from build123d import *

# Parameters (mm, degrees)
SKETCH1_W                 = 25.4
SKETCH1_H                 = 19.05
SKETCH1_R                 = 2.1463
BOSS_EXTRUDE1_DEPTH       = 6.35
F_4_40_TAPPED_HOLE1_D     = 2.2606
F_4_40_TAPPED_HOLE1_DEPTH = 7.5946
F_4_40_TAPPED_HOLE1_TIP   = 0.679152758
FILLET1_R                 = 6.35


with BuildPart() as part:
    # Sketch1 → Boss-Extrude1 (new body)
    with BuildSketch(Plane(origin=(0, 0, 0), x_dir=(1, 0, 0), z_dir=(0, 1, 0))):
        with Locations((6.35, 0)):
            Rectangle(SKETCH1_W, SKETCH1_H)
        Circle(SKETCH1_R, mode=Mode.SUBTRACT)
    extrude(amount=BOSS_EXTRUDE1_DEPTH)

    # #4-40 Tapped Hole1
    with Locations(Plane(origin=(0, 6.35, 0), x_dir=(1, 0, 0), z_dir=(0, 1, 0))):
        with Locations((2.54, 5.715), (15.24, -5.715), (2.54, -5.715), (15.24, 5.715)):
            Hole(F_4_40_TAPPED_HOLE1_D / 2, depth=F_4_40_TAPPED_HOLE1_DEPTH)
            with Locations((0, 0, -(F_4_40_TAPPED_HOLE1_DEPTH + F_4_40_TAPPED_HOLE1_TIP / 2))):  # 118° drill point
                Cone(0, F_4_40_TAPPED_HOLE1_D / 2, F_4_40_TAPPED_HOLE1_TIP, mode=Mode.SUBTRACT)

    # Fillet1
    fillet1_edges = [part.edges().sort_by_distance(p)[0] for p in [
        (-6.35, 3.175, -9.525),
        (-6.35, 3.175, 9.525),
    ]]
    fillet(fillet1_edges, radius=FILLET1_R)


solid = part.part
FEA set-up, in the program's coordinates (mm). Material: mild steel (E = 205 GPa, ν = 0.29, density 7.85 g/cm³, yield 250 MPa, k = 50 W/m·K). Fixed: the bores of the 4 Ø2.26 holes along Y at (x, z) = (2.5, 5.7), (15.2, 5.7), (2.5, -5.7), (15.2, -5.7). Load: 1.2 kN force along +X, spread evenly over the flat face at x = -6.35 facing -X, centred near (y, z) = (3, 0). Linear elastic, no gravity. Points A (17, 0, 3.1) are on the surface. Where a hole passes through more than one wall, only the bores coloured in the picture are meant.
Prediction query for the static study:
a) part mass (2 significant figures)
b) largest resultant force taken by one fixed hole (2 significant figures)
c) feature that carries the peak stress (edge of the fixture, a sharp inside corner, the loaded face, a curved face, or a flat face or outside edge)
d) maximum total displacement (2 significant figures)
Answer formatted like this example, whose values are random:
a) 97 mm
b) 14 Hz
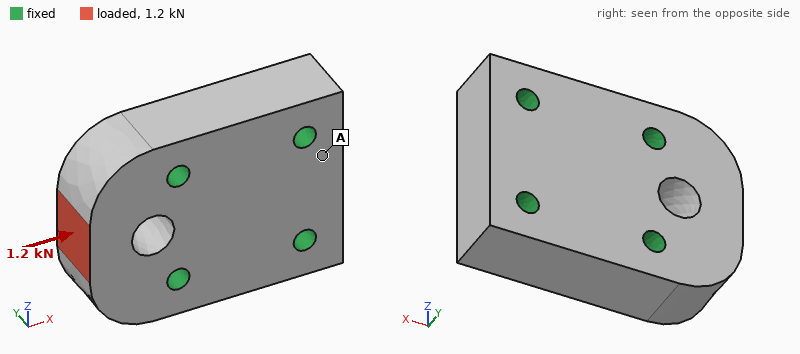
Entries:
a) 22 g
b) 610 N
c) a curved face
d) 1.5 µm
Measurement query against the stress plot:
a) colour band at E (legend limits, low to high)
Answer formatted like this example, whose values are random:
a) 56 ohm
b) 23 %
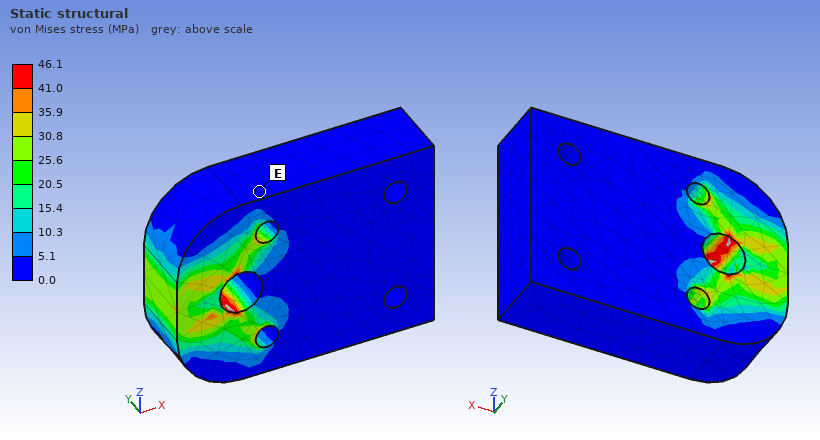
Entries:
a) 0.0 to 5.1 MPa
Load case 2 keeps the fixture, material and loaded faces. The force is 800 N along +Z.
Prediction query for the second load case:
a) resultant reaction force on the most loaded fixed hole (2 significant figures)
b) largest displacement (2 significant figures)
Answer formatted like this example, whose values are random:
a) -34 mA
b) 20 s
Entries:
a) 600 N
b) 1.6 µm
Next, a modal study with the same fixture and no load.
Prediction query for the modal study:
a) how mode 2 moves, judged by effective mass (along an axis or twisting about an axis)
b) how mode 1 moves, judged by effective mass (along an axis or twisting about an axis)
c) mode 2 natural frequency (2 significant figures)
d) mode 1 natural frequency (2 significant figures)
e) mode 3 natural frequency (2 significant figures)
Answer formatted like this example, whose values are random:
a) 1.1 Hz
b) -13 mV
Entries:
a) along Z
b) along Y
c) 70 kHz
d) 50 kHz
e) 79 kHz
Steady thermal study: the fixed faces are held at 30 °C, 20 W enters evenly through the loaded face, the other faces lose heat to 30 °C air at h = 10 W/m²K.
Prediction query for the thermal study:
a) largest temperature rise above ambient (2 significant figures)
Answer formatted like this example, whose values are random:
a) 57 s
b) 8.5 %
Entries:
a) 57 K
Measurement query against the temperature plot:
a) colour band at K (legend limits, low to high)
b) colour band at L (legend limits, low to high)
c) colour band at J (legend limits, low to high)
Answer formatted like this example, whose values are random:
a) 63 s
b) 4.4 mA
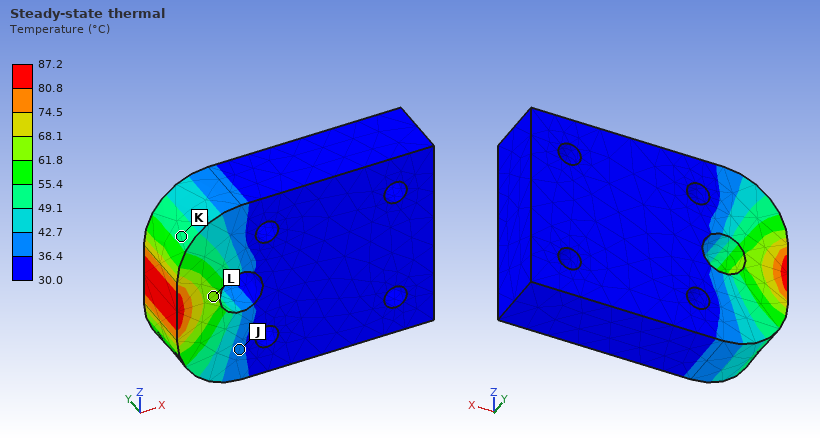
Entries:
a) 49.1 to 55.4 °C
b) 61.8 to 68.1 °C
c) 36.4 to 42.7 °C
